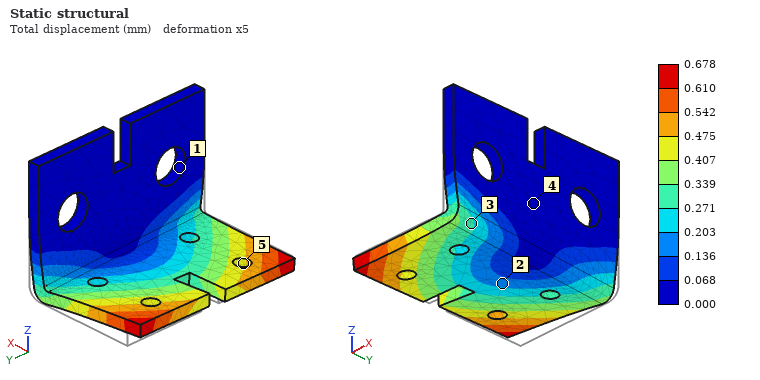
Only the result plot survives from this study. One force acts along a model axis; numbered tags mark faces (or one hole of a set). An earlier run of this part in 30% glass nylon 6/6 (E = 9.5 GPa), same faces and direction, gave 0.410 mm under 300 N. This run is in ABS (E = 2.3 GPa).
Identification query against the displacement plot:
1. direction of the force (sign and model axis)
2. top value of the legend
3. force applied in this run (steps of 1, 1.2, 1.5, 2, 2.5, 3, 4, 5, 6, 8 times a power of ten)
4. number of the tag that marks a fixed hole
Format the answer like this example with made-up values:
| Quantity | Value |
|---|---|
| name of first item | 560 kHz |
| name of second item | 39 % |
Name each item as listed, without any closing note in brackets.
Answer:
| Quantity | Value |
|---|---|
| direction of the force | -Y |
| top value of the legend | 0.678 mm |
| force applied in this run | 120 N |
| number of the tag that marks a fixed hole | 1 |
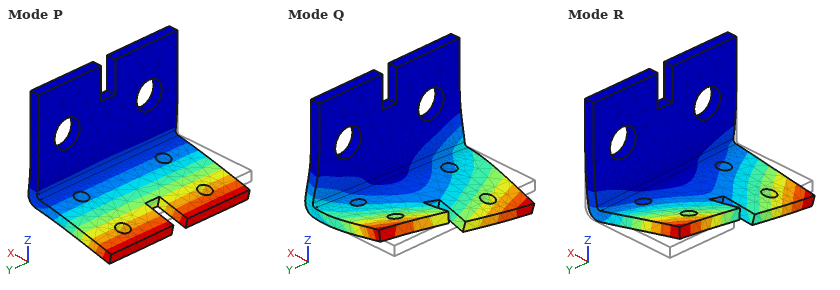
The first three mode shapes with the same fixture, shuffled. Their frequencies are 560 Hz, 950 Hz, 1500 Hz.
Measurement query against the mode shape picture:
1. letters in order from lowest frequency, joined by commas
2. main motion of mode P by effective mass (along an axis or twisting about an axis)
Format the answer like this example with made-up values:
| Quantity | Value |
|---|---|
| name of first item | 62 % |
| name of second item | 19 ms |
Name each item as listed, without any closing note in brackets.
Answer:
| Quantity | Value |
|---|---|
| letters in order from lowest frequency, joined by commas | P, R, Q |
| main motion of mode P by effective mass | along Z |
